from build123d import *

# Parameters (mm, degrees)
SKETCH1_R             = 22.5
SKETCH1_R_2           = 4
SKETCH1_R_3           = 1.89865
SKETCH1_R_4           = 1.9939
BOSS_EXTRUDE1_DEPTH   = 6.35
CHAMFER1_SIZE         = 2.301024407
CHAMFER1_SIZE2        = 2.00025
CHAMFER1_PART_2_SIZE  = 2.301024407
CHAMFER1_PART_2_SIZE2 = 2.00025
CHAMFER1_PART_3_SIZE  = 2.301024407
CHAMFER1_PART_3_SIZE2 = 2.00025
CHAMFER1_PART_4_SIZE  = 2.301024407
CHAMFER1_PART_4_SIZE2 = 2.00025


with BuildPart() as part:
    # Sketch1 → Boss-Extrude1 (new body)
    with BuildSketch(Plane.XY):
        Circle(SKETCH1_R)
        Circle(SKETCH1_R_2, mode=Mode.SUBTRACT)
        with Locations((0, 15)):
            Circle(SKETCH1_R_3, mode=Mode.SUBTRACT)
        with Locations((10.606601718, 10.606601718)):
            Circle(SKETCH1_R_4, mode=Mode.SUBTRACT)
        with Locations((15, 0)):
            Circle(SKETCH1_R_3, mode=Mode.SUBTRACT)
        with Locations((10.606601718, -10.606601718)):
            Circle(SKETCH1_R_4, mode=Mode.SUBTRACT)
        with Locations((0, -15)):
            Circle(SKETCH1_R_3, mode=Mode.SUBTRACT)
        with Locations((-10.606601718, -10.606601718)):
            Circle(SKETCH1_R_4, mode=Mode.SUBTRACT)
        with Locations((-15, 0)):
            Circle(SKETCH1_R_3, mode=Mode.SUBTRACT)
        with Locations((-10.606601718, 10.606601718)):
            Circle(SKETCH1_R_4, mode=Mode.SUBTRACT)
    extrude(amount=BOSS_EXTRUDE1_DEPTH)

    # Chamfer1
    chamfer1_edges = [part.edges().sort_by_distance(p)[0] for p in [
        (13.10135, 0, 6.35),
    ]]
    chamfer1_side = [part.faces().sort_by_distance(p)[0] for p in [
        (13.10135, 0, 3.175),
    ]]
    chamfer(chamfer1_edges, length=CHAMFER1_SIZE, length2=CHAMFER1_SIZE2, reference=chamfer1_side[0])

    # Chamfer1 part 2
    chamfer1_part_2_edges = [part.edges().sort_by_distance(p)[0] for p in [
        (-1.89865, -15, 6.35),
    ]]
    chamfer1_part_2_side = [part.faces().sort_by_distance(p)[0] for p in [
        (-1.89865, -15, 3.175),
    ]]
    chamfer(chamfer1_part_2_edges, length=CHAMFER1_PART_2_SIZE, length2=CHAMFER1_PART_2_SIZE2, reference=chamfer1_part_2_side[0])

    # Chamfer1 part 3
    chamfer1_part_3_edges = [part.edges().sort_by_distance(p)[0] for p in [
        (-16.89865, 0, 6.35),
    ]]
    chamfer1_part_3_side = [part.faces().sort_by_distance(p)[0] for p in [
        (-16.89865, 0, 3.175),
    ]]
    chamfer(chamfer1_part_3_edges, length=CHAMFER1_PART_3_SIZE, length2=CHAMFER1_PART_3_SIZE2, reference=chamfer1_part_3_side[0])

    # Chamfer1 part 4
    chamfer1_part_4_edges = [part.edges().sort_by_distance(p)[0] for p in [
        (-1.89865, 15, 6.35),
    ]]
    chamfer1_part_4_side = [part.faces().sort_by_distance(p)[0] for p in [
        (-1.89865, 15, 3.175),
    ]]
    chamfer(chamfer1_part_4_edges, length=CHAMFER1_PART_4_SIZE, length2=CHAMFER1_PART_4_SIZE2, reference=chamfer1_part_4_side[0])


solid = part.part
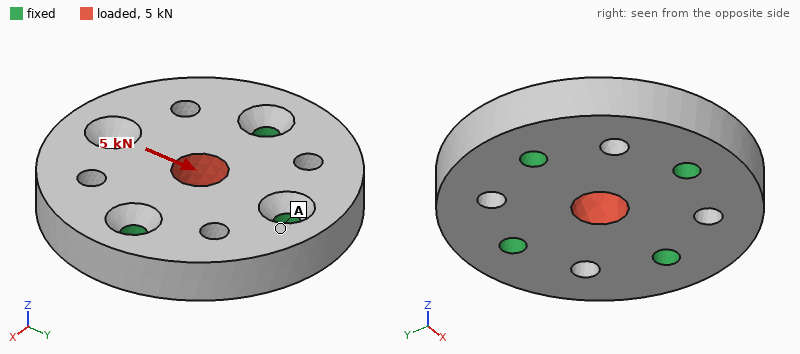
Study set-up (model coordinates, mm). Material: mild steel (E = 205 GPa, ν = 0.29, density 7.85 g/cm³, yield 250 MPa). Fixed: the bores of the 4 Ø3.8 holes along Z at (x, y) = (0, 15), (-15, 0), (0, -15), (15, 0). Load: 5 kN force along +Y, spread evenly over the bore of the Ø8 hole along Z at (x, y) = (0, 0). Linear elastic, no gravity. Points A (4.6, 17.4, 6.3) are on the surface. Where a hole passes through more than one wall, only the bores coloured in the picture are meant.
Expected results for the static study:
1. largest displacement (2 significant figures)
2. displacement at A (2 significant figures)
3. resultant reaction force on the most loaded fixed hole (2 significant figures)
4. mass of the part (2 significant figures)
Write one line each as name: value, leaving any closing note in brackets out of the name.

largest displacement: 1.9 µm
displacement at A: 0.56 µm
resultant reaction force on the most loaded fixed hole: 1.6 kN
mass of the part: 71 g
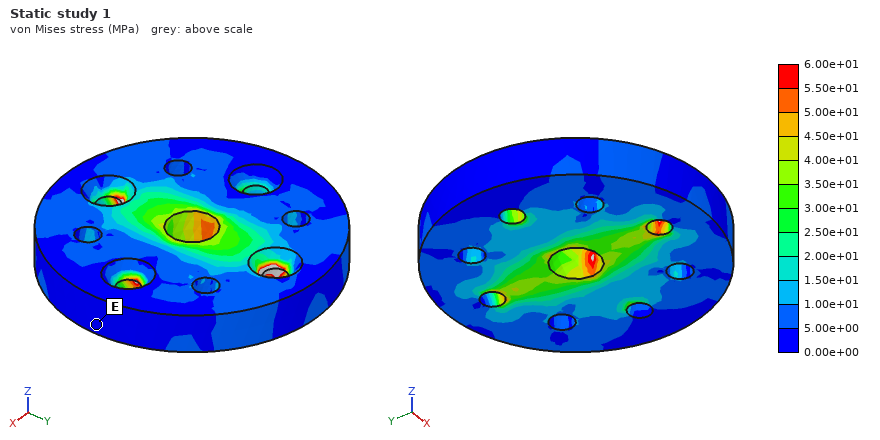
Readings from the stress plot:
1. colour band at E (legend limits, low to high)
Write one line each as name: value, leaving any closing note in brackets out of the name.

colour band at E: 0.00e+00 to 5.00e+00 MPa
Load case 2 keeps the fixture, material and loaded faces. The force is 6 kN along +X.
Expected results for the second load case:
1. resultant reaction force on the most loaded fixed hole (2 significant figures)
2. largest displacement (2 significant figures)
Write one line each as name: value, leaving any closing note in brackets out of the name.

resultant reaction force on the most loaded fixed hole: 2.0 kN
largest displacement: 2.2 µm
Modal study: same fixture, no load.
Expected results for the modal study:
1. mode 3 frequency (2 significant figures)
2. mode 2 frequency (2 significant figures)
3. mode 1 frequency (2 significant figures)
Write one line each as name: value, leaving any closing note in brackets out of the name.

mode 3 frequency: 27 kHz
mode 2 frequency: 27 kHz
mode 1 frequency: 24 kHz
